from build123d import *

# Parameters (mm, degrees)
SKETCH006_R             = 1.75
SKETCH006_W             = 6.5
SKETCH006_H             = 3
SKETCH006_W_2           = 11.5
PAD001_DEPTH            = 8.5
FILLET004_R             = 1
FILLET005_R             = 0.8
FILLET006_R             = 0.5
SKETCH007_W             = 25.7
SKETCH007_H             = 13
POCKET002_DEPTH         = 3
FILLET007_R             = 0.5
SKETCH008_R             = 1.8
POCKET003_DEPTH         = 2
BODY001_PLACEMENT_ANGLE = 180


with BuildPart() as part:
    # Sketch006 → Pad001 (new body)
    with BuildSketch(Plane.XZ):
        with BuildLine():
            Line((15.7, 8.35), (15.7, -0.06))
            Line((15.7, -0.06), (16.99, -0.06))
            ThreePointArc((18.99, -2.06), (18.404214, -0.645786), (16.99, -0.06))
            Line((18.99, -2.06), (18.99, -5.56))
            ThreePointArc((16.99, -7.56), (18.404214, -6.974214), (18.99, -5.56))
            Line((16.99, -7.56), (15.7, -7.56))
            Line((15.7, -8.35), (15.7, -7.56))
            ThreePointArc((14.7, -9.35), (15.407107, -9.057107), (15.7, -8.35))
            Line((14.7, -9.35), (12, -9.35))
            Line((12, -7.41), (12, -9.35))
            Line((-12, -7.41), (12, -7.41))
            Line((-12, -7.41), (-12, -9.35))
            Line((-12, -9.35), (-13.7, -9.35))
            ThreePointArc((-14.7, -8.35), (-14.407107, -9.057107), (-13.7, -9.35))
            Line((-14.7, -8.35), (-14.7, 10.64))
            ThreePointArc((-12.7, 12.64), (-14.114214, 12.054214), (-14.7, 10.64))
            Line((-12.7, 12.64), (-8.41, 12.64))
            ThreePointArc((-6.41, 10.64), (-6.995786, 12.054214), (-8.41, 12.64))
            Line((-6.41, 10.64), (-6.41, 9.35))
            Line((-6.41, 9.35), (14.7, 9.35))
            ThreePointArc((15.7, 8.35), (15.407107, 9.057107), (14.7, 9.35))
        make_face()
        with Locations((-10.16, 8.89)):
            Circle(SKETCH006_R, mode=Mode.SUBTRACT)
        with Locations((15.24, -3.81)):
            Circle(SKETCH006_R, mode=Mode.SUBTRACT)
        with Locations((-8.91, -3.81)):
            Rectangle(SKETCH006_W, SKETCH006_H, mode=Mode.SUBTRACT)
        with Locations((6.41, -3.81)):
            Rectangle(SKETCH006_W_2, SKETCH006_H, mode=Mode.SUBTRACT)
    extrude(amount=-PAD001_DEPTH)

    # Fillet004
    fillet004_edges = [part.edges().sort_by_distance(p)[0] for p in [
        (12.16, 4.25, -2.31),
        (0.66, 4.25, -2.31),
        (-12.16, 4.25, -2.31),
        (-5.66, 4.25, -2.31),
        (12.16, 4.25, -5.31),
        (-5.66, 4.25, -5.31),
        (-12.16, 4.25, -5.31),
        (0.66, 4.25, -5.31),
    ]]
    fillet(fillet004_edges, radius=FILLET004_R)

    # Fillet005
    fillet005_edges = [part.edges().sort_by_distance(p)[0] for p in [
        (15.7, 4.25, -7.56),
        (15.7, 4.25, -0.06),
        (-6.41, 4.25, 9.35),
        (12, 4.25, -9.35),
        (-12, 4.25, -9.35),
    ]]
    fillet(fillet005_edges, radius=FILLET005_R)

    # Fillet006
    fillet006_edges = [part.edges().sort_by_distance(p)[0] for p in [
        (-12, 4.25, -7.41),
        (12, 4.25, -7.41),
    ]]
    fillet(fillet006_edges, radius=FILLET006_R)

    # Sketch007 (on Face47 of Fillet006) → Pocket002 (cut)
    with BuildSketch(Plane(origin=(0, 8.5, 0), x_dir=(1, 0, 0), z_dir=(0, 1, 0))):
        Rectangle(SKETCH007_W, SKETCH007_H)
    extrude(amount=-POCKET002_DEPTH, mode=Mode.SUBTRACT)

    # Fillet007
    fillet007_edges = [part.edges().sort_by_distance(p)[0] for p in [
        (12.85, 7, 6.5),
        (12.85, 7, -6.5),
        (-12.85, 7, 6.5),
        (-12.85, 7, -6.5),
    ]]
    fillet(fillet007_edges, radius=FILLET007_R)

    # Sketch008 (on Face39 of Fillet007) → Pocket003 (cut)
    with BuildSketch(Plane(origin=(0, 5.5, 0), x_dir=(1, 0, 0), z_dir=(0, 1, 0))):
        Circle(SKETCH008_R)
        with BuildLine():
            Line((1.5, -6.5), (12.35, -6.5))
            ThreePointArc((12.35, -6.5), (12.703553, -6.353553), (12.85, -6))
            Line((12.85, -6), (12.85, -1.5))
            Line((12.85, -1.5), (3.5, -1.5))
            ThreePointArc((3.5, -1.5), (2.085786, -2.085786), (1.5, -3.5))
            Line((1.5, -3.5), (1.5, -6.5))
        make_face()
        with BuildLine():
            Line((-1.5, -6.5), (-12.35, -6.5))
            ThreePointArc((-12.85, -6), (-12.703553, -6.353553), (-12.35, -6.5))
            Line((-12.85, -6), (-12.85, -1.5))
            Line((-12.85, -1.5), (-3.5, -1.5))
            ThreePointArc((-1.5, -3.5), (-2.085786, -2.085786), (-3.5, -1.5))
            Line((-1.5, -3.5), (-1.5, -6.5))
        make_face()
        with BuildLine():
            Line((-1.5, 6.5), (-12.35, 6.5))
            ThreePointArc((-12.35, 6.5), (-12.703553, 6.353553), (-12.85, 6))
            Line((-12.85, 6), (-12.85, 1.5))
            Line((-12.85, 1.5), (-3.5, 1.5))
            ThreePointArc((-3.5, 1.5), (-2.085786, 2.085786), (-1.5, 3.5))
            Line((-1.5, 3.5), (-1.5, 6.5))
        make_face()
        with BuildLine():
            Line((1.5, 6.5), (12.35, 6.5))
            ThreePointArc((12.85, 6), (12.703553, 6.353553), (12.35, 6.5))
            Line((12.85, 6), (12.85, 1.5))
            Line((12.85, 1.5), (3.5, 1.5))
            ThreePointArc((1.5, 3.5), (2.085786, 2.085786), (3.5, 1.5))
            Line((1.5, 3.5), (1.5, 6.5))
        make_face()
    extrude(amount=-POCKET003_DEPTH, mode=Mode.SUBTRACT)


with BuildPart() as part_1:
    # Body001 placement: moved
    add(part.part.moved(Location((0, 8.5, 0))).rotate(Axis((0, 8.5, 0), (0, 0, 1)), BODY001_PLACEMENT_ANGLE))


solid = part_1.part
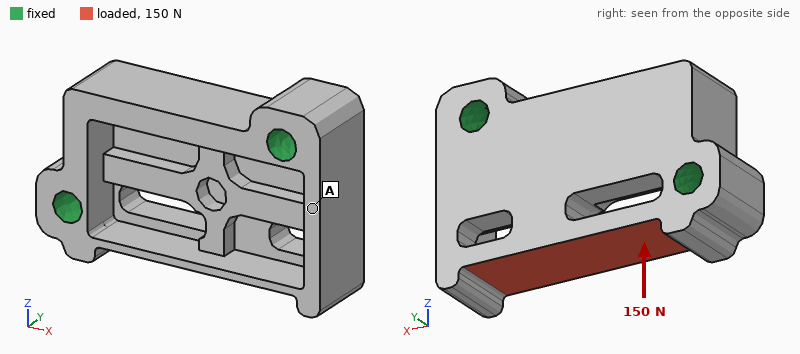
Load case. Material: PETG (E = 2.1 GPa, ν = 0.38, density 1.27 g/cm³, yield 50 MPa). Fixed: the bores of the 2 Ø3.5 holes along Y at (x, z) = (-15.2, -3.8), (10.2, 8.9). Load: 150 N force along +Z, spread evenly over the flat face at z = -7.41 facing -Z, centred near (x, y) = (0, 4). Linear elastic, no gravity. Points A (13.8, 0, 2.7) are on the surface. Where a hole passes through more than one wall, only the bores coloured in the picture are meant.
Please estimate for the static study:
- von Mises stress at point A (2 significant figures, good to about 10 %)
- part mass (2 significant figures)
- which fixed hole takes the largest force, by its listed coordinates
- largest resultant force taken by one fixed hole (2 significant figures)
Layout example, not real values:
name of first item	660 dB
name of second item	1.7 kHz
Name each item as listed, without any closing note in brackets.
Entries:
von Mises stress at point A	3.5 MPa
part mass	3.8 g
which fixed hole takes the largest force, by its listed coordinates	(10.2, 8.9)
largest resultant force taken by one fixed hole	96 N
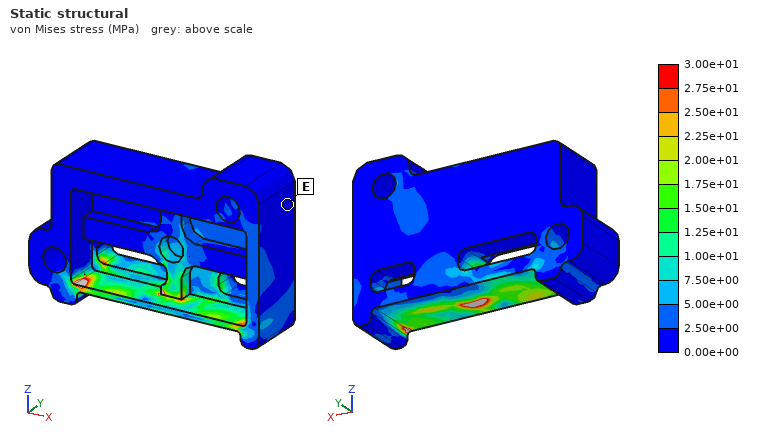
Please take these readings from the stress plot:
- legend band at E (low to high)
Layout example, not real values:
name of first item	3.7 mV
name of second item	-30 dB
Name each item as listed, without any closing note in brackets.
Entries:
legend band at E	0.00e+00 to 2.50e+00 MPa
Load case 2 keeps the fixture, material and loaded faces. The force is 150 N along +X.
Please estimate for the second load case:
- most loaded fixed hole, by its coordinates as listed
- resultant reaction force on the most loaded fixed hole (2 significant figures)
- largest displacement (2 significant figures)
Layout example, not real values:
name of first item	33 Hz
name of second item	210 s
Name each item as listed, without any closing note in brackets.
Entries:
most loaded fixed hole, by its coordinates as listed	(-15.2, -3.8)
resultant reaction force on the most loaded fixed hole	120 N
largest displacement	86 µm
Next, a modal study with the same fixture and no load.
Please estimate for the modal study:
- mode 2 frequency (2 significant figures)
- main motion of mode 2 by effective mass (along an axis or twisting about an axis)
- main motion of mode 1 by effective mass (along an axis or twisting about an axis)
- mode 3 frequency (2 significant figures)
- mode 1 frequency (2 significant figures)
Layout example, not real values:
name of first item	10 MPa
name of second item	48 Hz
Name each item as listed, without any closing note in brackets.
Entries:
mode 2 frequency	7000 Hz
main motion of mode 2 by effective mass	along Y
main motion of mode 1 by effective mass	along Y
mode 3 frequency	7700 Hz
mode 1 frequency	4300 Hz
